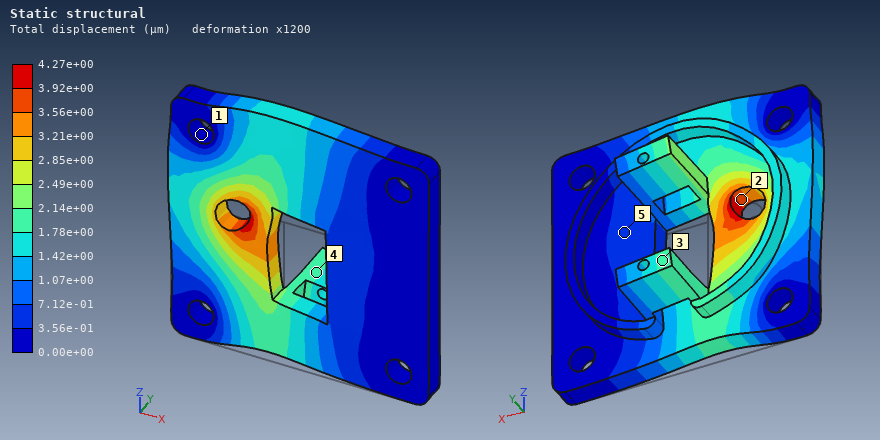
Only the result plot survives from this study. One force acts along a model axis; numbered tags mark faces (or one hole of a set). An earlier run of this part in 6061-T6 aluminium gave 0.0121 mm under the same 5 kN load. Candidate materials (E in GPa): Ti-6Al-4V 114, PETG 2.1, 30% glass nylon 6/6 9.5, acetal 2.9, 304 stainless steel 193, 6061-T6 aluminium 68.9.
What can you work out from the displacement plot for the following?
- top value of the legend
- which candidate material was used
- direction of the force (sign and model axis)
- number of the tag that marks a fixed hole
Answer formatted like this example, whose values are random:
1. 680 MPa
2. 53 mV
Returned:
1. 4.27e+00 µm
2. 304 stainless steel
3. +Z
4. 1
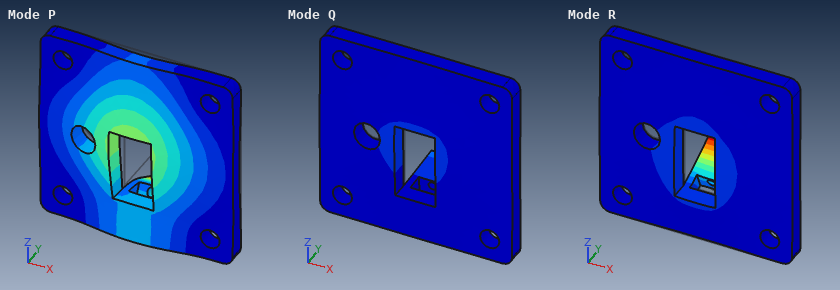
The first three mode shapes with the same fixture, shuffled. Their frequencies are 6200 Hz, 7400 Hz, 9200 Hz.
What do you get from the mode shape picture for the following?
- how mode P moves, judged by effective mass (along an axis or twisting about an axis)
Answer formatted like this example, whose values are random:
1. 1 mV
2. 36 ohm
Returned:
1. along Y
